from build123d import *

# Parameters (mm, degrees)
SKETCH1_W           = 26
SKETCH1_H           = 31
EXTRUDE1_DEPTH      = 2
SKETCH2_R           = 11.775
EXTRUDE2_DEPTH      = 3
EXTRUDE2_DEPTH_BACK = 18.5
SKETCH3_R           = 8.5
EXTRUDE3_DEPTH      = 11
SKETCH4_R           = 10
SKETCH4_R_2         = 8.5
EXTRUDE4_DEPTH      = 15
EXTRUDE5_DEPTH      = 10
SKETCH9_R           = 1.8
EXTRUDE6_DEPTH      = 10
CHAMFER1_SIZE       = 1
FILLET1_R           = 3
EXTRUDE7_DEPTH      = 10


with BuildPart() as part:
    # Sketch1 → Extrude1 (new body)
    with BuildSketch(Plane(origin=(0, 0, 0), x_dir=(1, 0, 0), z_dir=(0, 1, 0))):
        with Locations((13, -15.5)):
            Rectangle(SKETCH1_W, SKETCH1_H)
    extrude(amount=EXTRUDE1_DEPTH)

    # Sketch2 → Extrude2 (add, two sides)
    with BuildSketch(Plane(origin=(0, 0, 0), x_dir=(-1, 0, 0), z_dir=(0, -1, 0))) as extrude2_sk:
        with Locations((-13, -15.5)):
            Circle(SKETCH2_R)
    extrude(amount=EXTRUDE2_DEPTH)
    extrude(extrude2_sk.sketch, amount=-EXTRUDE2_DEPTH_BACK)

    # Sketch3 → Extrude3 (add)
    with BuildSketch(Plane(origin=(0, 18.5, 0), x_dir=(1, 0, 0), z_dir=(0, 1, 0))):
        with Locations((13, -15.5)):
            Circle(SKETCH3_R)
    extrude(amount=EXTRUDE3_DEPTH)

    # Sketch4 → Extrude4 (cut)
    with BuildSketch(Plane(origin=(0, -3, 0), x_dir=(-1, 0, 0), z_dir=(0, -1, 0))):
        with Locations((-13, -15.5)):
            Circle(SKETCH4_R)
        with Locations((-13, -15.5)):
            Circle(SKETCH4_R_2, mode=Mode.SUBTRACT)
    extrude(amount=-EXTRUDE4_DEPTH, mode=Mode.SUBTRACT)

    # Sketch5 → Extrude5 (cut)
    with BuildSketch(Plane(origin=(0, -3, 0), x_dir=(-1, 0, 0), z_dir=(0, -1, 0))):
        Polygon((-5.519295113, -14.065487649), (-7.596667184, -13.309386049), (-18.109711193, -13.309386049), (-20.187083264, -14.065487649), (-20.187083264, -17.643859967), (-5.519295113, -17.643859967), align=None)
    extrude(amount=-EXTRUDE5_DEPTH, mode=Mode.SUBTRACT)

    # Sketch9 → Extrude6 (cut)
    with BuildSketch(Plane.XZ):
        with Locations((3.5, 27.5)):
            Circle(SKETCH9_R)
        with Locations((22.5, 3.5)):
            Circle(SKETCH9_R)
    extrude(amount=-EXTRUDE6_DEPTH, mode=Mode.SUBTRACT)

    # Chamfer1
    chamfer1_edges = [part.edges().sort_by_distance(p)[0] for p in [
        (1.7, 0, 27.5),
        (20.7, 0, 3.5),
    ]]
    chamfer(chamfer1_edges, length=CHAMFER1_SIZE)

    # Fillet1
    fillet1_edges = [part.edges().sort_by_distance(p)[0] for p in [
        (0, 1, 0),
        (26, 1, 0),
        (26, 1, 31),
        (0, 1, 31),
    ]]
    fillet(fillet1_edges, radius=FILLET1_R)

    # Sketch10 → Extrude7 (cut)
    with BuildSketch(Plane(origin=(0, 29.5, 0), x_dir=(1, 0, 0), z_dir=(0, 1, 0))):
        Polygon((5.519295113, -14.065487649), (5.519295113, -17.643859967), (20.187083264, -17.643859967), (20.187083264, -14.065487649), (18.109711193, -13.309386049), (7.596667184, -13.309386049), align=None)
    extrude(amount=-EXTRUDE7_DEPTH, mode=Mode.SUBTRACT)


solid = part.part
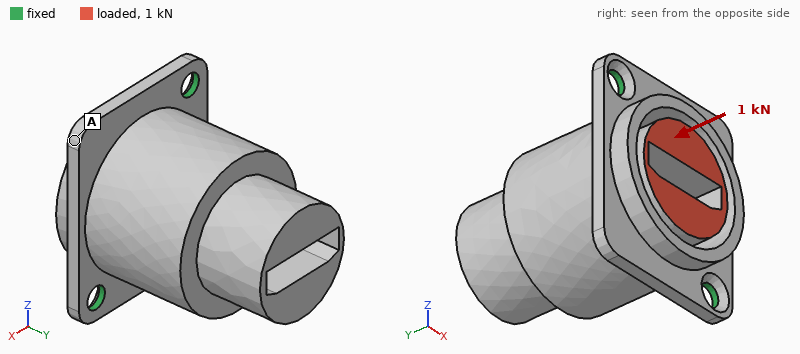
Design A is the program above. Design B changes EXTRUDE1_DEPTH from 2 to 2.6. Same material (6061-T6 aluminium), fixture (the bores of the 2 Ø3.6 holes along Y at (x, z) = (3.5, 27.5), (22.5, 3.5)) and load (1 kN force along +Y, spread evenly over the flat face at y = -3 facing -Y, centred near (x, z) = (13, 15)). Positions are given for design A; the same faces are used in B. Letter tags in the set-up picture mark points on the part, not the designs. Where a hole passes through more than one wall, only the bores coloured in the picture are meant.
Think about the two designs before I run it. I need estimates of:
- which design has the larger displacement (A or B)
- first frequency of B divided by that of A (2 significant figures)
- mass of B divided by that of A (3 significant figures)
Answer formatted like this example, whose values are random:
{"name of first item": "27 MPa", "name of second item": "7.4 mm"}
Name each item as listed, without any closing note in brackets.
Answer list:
{"which design has the larger displacement": "A", "first frequency of B divided by that of A": "1.4", "mass of B divided by that of A": "1.02"}
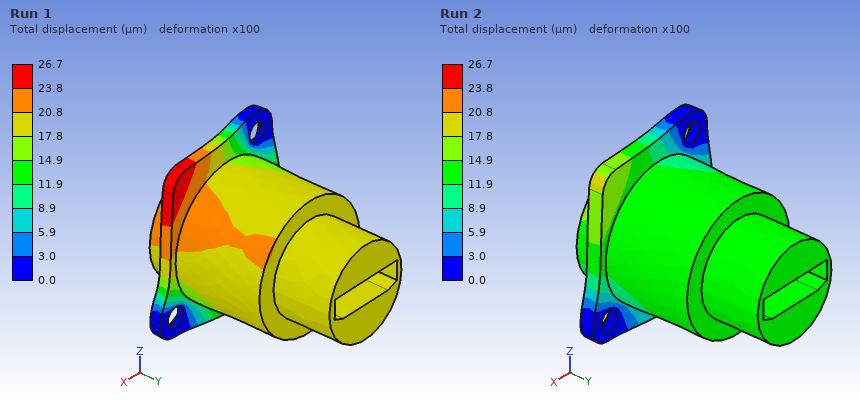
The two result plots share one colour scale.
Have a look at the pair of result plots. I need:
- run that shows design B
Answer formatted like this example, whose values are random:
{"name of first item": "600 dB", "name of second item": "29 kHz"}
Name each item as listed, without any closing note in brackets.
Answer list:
{"run that shows design B": "Run 2"}
